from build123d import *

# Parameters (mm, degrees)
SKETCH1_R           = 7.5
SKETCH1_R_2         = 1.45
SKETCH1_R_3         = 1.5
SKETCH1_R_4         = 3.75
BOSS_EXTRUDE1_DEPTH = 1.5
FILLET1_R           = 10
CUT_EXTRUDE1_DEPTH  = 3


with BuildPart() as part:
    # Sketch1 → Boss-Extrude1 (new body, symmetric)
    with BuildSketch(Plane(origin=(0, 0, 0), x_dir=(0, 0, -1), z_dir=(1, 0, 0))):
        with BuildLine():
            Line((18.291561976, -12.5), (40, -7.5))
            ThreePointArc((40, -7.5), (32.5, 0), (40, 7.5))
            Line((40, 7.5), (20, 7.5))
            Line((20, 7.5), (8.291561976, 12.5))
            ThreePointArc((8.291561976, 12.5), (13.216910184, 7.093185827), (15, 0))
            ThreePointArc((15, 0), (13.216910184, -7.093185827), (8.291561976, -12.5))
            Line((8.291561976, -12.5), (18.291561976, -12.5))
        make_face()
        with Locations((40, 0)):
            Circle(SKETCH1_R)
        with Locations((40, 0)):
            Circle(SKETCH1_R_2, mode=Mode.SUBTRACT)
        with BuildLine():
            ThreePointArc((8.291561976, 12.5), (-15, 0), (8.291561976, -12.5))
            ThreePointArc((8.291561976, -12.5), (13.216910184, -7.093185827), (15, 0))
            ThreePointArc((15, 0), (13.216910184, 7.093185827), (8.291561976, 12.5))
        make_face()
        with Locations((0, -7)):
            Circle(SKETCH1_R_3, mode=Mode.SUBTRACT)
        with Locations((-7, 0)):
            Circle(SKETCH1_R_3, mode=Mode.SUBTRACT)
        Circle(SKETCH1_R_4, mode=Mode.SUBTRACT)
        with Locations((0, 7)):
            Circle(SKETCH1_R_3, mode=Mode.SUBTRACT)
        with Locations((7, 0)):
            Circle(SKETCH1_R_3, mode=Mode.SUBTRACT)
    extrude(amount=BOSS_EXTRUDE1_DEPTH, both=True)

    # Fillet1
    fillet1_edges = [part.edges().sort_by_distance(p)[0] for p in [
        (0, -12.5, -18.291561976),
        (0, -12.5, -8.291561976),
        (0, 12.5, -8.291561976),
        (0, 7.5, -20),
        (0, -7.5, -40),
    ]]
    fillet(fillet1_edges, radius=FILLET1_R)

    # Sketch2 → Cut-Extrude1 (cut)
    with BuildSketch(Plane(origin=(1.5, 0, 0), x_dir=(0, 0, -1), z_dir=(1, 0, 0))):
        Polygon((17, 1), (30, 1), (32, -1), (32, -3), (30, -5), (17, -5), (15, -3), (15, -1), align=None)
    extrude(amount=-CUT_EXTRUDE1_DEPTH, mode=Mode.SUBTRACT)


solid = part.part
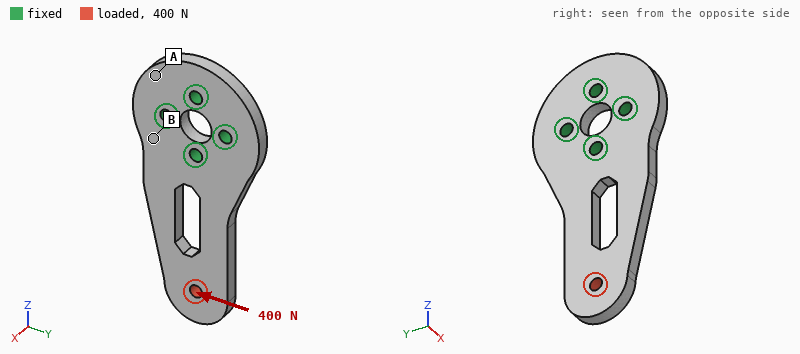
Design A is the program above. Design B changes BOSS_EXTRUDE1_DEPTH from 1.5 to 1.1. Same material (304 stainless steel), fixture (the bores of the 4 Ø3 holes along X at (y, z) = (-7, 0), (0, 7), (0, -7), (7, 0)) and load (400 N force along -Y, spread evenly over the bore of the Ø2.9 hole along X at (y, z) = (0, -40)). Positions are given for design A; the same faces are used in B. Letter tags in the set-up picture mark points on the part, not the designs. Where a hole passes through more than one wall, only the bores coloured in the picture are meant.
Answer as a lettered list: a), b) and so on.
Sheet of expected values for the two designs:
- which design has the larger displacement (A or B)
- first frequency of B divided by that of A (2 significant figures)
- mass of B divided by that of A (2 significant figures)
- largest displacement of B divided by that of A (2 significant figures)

a) B
b) 0.74
c) 0.73
d) 1.4
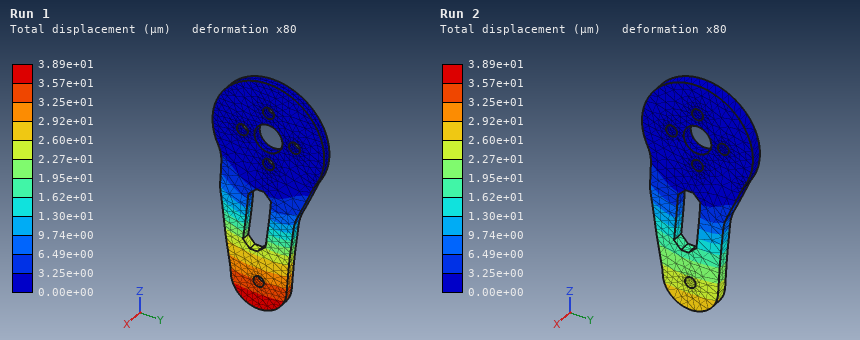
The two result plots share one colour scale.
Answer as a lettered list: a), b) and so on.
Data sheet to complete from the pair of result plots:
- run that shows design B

a) Run 1
